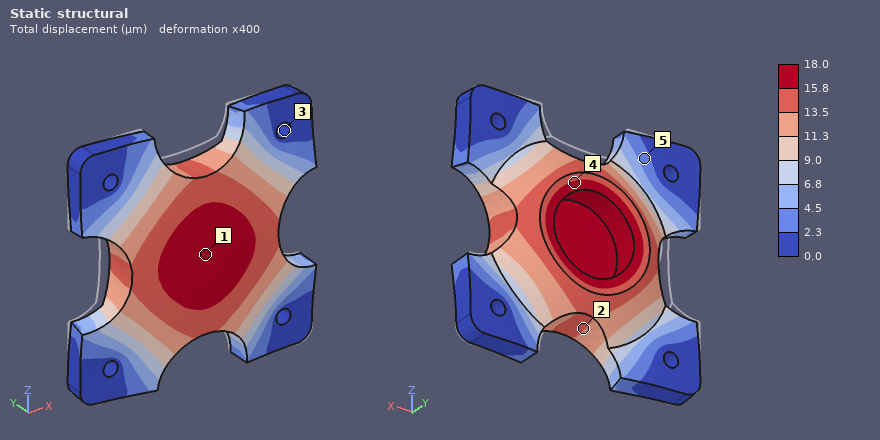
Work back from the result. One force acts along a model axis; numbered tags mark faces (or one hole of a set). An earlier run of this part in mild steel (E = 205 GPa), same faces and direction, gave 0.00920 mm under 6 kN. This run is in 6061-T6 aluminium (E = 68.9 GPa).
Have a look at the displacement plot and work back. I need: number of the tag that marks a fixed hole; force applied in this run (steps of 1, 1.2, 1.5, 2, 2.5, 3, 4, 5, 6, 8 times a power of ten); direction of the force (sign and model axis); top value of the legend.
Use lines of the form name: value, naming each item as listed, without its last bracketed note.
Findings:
number of the tag that marks a fixed hole: 3
force applied in this run: 4 kN
direction of the force: -Y
top value of the legend: 18.0 µm
